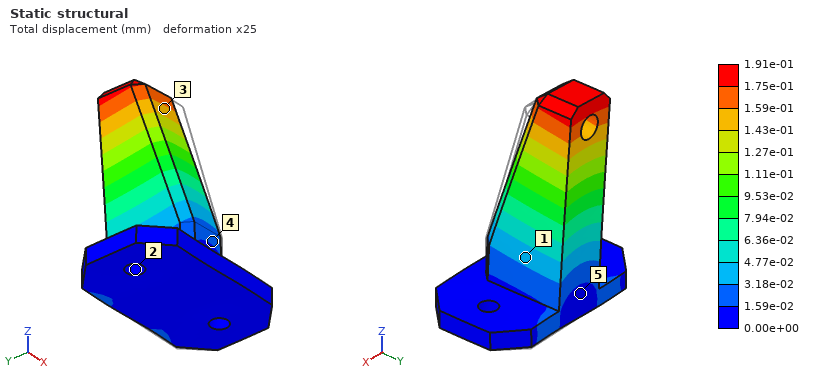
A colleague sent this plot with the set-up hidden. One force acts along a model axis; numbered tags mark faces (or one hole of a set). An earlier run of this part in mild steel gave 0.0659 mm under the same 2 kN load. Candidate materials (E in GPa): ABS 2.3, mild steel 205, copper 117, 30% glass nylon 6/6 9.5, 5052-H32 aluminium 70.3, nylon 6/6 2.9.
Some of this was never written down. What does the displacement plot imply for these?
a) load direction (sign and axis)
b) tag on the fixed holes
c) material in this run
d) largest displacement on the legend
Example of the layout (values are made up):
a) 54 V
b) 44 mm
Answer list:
a) -X
b) 2
c) 5052-H32 aluminium
d) 1.91e-01 mm
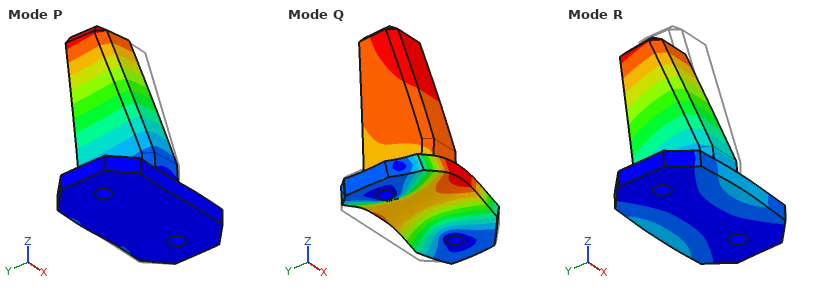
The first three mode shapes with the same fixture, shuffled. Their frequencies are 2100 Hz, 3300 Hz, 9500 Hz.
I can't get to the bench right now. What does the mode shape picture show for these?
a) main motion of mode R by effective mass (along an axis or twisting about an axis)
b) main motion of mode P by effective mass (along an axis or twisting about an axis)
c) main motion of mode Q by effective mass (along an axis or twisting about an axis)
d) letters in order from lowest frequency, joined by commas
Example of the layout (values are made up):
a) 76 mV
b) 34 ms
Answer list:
a) along Y
b) along X
c) along Z
d) R, P, Q
